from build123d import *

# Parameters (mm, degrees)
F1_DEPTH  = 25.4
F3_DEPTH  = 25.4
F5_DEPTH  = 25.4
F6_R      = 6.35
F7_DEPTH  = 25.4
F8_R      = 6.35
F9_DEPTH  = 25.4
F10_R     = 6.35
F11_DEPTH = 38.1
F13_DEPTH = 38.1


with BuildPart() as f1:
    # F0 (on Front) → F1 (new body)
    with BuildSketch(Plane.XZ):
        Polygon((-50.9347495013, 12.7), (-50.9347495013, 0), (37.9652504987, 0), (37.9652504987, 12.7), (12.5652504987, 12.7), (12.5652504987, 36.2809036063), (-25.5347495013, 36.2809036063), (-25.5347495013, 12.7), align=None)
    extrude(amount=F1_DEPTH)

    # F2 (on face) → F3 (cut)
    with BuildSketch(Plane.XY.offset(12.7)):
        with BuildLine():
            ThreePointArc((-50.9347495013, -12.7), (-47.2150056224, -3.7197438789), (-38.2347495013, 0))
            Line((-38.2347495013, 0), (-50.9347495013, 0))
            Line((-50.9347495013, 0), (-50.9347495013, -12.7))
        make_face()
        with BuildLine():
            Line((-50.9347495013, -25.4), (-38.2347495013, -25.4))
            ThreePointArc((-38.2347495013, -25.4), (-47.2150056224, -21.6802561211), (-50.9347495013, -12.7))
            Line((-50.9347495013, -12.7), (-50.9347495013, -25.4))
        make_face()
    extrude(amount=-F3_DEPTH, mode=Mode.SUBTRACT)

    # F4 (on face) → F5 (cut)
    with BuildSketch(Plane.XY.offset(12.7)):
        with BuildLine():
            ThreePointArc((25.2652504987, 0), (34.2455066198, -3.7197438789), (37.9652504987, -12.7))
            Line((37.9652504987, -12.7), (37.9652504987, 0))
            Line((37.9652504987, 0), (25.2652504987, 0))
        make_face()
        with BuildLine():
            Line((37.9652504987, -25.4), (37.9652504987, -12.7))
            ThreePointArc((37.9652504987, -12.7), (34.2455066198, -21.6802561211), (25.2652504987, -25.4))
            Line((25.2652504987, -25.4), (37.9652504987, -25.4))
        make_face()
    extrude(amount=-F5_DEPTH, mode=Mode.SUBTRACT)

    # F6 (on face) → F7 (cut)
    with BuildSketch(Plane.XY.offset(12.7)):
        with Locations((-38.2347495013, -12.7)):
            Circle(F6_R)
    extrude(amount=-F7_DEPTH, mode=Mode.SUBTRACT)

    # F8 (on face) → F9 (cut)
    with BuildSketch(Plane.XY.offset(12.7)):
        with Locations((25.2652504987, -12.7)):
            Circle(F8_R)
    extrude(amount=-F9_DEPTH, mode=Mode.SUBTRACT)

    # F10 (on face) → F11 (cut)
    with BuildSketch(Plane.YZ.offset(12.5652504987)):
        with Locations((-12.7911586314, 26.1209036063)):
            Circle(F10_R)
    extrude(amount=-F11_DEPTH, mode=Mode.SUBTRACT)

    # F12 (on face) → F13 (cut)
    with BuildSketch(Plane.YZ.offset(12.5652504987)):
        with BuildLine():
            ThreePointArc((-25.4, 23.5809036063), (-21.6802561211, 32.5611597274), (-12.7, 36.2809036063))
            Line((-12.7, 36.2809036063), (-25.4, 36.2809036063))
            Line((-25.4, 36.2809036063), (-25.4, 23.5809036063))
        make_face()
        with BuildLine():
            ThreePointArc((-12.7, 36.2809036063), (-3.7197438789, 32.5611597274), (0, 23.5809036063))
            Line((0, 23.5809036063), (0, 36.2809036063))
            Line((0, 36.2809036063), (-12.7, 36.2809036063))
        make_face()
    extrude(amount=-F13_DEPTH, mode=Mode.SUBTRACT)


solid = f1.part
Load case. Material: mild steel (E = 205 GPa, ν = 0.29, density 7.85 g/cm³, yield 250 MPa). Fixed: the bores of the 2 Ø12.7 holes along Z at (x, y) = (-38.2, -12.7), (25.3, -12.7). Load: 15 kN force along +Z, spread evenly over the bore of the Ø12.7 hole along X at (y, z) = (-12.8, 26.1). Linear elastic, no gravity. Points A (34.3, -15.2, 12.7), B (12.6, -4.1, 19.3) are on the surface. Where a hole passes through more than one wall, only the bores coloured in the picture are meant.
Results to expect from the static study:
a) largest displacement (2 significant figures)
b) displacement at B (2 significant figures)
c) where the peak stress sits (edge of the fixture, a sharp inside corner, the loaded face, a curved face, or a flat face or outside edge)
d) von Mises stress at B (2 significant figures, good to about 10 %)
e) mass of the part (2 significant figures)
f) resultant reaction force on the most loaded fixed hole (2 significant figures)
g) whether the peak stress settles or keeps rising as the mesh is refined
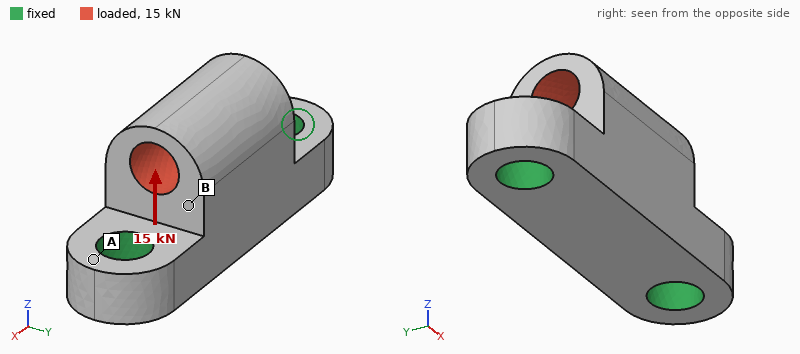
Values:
11 µm
7.2 µm
edge of the fixture
40 MPa
310 g
8.0 kN
keeps rising
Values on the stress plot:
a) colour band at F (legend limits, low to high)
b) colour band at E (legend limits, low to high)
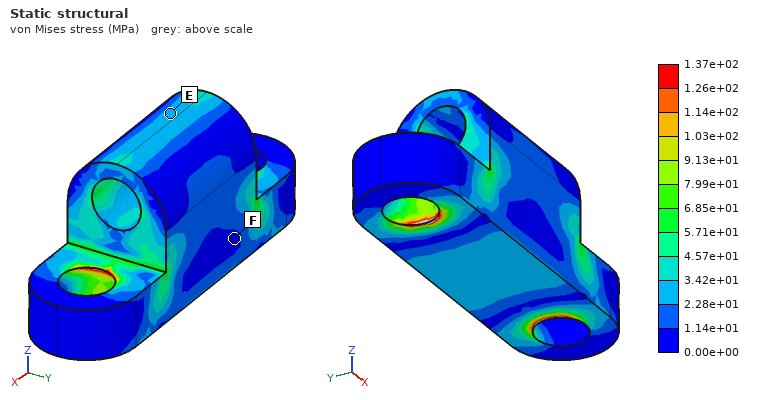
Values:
0.00e+00 to 1.14e+01 MPa
2.28e+01 to 3.42e+01 MPa
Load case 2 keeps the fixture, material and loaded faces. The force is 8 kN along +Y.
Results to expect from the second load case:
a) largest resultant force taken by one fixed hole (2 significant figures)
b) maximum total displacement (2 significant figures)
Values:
4.0 kN
37 µm
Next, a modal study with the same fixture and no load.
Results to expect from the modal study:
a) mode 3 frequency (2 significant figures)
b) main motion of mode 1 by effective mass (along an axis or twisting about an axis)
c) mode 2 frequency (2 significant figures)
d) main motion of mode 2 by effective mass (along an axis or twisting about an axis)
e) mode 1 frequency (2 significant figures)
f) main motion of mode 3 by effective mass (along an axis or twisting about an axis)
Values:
18 kHz
along Y
15 kHz
along Z
8300 Hz
along X
